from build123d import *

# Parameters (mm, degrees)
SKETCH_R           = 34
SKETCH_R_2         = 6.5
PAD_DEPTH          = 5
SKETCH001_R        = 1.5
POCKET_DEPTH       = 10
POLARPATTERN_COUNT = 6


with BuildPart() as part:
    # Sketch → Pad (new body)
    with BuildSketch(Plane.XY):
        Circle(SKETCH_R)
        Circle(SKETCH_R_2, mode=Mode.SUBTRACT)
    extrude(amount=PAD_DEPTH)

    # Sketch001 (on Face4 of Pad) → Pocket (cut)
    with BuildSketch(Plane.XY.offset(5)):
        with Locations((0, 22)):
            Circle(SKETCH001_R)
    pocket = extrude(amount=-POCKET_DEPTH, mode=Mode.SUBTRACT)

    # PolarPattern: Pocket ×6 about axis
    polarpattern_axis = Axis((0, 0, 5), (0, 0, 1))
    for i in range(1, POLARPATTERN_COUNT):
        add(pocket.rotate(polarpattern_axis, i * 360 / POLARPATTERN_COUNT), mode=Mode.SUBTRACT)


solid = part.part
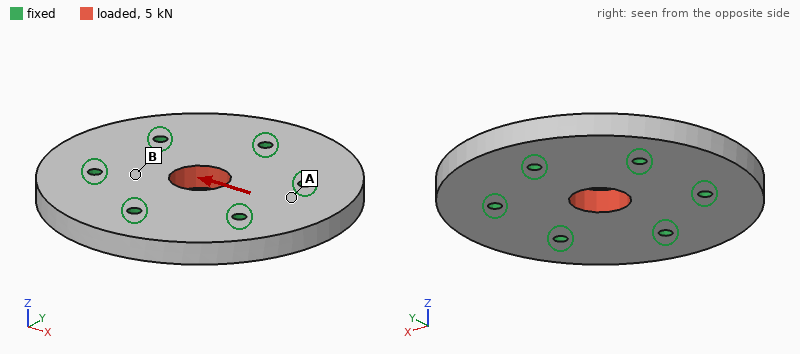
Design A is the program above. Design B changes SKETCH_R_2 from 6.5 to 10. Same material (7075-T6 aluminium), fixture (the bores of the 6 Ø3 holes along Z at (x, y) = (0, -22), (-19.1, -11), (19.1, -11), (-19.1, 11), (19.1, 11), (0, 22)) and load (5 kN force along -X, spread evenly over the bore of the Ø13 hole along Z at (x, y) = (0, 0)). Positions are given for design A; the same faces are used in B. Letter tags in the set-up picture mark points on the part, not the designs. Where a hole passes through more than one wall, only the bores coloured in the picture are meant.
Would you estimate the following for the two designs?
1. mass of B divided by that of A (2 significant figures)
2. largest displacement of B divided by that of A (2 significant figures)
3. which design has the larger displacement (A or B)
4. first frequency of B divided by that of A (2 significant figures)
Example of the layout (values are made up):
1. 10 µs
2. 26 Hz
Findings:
1. 0.95
2. 0.71
3. A
4. 1.0
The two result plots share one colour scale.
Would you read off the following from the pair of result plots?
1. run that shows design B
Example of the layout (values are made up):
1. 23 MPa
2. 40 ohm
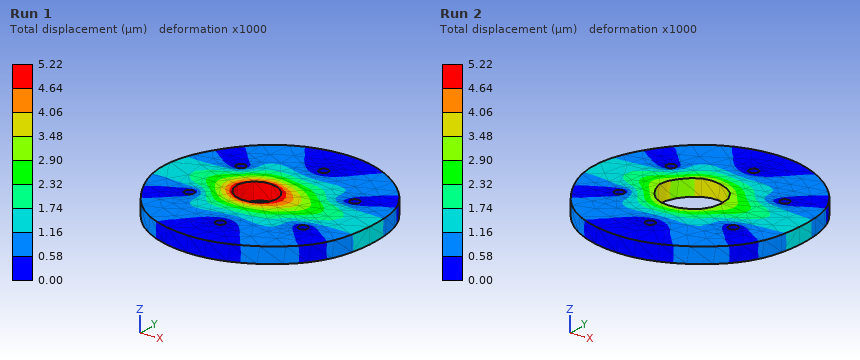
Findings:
1. Run 2
